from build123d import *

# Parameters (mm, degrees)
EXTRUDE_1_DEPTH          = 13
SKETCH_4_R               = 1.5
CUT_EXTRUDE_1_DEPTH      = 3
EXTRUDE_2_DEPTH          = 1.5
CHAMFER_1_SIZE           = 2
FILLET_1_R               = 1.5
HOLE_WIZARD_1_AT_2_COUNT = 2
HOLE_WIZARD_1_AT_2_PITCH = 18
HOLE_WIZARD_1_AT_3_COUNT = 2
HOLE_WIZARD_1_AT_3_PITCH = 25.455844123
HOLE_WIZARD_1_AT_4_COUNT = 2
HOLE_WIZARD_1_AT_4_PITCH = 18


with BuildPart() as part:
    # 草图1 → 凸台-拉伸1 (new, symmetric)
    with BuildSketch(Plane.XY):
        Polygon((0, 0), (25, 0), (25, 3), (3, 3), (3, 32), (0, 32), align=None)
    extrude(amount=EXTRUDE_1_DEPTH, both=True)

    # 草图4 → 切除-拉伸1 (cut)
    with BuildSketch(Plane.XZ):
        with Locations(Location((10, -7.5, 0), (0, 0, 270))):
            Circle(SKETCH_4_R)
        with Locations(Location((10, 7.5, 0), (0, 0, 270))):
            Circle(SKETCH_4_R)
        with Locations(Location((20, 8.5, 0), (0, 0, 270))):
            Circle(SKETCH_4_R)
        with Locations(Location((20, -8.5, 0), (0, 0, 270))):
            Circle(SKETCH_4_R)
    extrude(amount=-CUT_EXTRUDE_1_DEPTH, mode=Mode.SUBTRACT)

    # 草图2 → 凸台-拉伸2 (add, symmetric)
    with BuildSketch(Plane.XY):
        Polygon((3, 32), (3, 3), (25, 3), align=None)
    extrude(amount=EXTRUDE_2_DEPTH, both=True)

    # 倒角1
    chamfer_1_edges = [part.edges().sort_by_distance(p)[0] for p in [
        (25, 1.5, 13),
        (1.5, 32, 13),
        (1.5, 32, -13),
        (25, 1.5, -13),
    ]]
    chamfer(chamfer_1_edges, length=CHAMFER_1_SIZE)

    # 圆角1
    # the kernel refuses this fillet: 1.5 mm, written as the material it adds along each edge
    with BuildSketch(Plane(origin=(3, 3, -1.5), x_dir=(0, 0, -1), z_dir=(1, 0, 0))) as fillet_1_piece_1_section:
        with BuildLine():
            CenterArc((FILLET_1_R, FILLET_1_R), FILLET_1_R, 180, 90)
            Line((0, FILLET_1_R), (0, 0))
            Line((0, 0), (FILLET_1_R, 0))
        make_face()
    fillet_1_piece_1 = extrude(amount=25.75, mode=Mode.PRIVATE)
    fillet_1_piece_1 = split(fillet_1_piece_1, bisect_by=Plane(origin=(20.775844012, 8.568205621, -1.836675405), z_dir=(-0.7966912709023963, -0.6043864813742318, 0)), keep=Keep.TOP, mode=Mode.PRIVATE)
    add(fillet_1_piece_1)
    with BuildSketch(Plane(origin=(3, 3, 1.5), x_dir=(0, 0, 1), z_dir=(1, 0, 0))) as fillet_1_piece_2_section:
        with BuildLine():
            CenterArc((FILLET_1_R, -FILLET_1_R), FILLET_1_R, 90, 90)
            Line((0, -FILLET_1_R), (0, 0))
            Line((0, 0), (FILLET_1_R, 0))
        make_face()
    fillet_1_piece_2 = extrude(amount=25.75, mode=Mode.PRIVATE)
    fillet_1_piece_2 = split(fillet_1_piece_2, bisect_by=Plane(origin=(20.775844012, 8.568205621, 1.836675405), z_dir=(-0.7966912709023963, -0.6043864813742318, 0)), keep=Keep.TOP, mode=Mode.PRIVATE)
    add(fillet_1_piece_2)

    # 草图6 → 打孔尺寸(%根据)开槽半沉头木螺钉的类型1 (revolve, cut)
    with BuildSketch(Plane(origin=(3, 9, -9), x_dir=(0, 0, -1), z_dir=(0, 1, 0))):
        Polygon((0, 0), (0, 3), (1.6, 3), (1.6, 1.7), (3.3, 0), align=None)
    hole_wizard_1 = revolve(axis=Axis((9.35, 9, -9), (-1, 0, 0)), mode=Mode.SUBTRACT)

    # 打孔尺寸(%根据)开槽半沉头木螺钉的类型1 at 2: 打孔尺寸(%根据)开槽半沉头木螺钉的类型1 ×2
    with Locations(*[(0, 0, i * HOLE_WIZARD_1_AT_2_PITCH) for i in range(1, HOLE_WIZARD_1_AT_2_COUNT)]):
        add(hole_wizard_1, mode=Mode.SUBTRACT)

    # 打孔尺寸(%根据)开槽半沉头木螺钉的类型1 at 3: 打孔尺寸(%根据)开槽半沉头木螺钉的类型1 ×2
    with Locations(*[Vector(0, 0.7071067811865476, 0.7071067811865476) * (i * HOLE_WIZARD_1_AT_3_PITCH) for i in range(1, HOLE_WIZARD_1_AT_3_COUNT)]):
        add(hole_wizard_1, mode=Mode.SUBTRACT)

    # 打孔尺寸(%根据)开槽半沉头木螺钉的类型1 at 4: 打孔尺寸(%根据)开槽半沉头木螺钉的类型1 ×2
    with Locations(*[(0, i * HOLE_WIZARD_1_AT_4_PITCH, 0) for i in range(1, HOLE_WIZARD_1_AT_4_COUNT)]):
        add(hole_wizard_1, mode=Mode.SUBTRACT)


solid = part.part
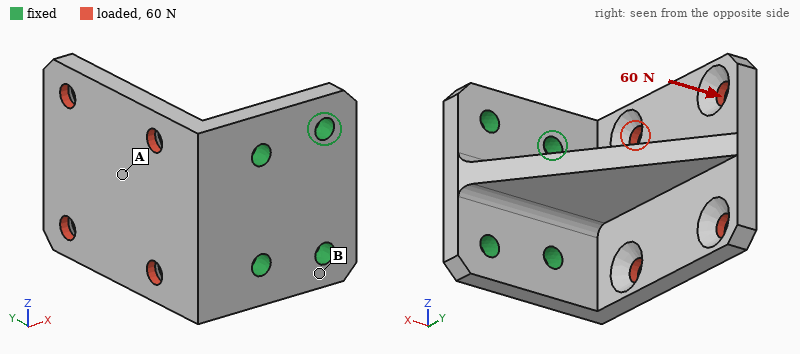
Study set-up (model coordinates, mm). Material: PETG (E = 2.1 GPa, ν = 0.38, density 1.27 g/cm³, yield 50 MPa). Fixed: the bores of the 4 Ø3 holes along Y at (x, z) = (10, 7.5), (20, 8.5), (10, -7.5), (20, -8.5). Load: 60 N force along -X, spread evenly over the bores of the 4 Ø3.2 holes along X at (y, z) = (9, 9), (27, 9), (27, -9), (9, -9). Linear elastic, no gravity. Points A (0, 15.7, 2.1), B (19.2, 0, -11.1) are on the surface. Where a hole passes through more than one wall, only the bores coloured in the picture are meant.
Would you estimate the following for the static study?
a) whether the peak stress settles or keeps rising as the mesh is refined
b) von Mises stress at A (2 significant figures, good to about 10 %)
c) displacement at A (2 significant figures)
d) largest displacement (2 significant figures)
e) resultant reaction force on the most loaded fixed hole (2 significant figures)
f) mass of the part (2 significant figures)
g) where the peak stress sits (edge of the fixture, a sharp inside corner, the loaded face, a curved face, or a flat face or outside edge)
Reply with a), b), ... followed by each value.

a) keeps rising
b) 3.0 MPa
c) 0.12 mm
d) 0.29 mm
e) 38 N
f) 6.2 g
g) edge of the fixture
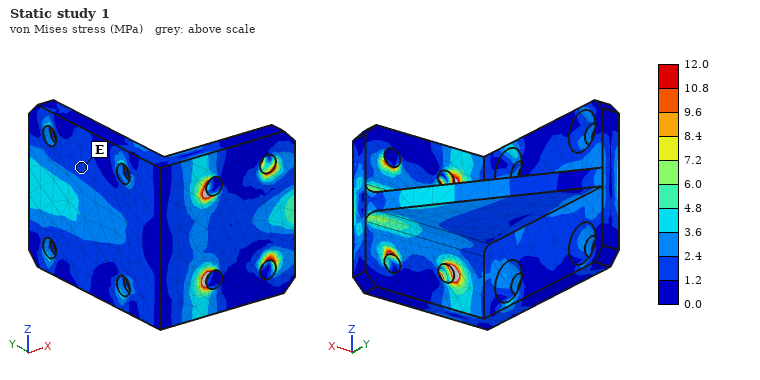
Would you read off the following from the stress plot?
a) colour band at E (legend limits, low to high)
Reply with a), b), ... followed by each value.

a) 1.2 to 2.4 MPa
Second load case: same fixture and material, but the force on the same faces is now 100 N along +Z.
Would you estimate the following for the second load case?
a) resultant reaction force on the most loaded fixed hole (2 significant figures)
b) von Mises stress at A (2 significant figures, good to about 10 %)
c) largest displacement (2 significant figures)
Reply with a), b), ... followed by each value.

a) 120 N
b) 3.4 MPa
c) 0.55 mm
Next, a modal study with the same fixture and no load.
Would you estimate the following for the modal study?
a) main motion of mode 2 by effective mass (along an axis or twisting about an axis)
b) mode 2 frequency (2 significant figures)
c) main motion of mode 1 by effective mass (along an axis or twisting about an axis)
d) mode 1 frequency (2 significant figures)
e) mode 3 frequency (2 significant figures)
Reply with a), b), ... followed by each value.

a) along X
b) 1600 Hz
c) along Z
d) 1400 Hz
e) 2100 Hz
